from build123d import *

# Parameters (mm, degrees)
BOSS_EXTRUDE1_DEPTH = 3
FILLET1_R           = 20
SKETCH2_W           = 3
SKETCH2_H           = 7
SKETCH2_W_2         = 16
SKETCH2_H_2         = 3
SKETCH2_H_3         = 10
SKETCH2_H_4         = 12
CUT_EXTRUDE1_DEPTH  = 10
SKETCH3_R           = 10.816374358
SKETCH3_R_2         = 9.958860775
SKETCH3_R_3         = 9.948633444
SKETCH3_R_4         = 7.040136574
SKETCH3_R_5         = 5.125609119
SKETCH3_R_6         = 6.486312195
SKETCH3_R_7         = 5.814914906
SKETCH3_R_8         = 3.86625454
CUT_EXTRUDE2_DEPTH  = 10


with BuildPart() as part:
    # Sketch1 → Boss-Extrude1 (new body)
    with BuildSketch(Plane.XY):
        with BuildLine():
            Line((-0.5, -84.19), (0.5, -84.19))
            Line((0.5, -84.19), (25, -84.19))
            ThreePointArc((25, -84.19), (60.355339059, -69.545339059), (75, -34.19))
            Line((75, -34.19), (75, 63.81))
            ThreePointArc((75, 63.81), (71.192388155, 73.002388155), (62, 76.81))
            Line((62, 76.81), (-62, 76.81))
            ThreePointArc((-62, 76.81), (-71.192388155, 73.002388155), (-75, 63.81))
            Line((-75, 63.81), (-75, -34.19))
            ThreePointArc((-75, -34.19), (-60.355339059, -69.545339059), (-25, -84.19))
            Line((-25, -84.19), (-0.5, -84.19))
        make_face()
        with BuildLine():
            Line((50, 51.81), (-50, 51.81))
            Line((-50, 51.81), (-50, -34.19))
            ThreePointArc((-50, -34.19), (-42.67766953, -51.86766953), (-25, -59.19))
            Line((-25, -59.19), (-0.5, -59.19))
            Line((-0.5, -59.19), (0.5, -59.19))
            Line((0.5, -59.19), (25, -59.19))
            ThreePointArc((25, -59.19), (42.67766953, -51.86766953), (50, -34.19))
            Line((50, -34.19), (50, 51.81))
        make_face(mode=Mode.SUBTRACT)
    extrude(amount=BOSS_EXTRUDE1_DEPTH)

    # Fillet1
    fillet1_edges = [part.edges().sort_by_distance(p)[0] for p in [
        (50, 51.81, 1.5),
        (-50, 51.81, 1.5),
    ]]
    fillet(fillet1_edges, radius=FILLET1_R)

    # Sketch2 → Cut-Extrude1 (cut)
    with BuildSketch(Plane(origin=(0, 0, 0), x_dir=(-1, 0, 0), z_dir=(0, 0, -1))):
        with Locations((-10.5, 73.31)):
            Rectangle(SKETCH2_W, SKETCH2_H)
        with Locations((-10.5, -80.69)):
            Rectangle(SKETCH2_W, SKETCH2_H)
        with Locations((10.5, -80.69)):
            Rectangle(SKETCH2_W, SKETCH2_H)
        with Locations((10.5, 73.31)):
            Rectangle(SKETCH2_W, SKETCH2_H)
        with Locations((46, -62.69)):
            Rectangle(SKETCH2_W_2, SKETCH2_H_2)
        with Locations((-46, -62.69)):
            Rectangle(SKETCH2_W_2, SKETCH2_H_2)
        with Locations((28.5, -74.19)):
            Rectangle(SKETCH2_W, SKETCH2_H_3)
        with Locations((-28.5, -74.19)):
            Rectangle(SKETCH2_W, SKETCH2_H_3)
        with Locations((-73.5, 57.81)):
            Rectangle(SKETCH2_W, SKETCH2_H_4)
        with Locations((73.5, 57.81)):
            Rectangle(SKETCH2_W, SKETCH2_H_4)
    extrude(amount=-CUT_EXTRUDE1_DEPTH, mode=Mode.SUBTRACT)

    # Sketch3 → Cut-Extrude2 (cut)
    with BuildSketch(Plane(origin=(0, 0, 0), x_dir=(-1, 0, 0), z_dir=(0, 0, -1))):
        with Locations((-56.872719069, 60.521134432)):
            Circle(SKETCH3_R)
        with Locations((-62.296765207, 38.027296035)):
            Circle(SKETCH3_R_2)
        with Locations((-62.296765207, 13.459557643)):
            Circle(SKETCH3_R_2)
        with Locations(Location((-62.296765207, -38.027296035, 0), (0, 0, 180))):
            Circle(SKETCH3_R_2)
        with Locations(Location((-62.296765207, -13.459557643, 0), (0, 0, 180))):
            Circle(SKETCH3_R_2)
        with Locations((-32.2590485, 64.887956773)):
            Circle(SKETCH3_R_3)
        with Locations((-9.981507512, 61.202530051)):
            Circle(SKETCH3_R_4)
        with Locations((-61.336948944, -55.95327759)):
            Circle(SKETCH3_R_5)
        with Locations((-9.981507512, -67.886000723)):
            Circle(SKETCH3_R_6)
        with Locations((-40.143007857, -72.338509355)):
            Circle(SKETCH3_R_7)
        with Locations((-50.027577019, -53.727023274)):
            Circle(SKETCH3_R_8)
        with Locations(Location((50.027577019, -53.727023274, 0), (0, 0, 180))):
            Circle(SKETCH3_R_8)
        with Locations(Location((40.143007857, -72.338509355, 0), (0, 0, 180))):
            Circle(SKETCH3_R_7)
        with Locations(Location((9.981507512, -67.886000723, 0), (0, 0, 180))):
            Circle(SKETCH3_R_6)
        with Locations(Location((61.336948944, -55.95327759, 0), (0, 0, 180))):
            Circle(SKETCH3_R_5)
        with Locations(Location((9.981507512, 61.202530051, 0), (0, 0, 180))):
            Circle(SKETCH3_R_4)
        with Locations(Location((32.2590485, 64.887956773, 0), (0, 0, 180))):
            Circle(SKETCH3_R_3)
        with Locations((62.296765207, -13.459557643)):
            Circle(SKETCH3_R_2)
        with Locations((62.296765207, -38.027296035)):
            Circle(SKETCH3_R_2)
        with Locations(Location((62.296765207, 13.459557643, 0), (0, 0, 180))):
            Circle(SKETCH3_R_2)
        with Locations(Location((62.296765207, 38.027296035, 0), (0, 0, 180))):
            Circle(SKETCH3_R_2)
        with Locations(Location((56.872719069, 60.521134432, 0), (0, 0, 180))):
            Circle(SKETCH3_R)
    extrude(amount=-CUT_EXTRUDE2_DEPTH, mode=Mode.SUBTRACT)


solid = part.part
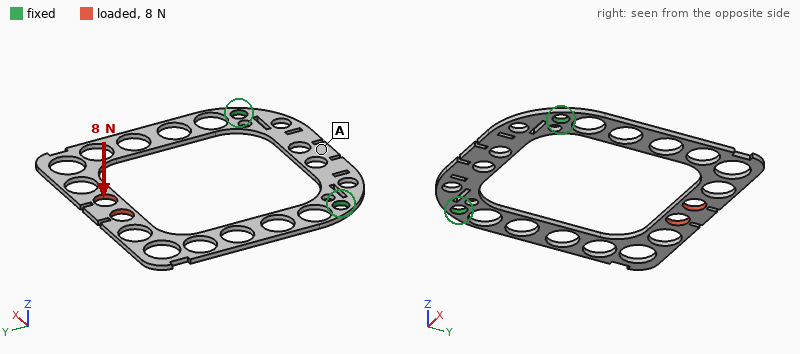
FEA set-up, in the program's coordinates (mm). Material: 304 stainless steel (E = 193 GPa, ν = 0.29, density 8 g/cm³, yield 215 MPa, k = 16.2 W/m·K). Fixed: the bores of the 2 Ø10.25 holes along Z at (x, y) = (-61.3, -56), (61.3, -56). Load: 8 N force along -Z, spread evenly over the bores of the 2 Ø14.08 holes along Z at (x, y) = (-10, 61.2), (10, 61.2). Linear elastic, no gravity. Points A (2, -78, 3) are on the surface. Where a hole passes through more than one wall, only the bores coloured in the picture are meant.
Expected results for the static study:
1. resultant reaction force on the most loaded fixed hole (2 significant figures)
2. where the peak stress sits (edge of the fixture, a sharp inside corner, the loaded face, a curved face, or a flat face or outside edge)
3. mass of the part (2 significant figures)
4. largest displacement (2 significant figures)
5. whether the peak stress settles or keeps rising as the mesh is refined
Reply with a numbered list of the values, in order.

1. 4.0 N
2. a sharp inside corner
3. 170 g
4. 0.70 mm
5. keeps rising
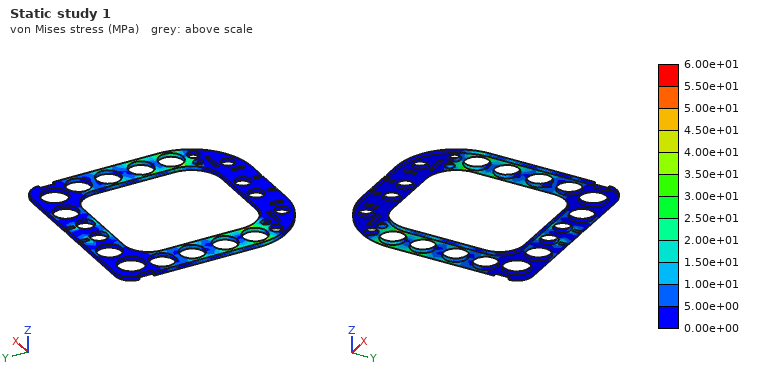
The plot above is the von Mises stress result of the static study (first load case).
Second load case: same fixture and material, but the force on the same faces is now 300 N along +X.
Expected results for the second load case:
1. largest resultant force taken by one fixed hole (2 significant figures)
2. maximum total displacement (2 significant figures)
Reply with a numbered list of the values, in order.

1. 230 N
2. 0.14 mm
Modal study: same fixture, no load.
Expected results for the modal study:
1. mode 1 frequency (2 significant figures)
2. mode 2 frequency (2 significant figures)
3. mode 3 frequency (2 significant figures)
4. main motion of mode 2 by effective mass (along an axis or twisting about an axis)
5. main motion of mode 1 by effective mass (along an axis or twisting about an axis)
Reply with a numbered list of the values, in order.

1. 75 Hz
2. 190 Hz
3. 510 Hz
4. twisting about Y
5. along Z
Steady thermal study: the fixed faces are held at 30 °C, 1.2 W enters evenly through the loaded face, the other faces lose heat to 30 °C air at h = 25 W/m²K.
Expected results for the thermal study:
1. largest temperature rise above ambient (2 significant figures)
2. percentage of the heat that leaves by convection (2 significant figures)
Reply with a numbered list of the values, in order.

1. 20 K
2. 100 %
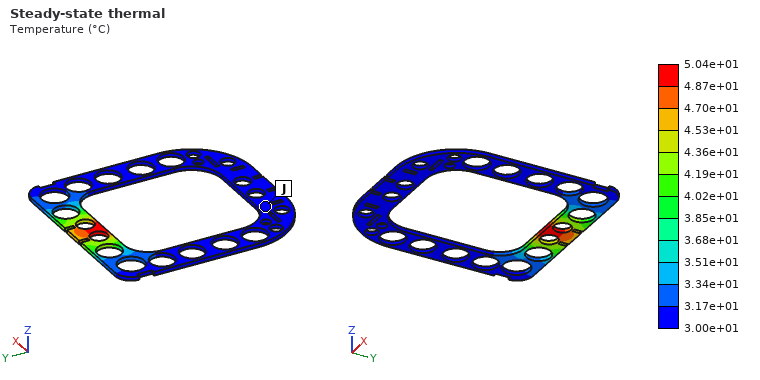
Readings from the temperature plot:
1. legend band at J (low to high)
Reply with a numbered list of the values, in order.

1. 3.00e+01 to 3.17e+01 °C
